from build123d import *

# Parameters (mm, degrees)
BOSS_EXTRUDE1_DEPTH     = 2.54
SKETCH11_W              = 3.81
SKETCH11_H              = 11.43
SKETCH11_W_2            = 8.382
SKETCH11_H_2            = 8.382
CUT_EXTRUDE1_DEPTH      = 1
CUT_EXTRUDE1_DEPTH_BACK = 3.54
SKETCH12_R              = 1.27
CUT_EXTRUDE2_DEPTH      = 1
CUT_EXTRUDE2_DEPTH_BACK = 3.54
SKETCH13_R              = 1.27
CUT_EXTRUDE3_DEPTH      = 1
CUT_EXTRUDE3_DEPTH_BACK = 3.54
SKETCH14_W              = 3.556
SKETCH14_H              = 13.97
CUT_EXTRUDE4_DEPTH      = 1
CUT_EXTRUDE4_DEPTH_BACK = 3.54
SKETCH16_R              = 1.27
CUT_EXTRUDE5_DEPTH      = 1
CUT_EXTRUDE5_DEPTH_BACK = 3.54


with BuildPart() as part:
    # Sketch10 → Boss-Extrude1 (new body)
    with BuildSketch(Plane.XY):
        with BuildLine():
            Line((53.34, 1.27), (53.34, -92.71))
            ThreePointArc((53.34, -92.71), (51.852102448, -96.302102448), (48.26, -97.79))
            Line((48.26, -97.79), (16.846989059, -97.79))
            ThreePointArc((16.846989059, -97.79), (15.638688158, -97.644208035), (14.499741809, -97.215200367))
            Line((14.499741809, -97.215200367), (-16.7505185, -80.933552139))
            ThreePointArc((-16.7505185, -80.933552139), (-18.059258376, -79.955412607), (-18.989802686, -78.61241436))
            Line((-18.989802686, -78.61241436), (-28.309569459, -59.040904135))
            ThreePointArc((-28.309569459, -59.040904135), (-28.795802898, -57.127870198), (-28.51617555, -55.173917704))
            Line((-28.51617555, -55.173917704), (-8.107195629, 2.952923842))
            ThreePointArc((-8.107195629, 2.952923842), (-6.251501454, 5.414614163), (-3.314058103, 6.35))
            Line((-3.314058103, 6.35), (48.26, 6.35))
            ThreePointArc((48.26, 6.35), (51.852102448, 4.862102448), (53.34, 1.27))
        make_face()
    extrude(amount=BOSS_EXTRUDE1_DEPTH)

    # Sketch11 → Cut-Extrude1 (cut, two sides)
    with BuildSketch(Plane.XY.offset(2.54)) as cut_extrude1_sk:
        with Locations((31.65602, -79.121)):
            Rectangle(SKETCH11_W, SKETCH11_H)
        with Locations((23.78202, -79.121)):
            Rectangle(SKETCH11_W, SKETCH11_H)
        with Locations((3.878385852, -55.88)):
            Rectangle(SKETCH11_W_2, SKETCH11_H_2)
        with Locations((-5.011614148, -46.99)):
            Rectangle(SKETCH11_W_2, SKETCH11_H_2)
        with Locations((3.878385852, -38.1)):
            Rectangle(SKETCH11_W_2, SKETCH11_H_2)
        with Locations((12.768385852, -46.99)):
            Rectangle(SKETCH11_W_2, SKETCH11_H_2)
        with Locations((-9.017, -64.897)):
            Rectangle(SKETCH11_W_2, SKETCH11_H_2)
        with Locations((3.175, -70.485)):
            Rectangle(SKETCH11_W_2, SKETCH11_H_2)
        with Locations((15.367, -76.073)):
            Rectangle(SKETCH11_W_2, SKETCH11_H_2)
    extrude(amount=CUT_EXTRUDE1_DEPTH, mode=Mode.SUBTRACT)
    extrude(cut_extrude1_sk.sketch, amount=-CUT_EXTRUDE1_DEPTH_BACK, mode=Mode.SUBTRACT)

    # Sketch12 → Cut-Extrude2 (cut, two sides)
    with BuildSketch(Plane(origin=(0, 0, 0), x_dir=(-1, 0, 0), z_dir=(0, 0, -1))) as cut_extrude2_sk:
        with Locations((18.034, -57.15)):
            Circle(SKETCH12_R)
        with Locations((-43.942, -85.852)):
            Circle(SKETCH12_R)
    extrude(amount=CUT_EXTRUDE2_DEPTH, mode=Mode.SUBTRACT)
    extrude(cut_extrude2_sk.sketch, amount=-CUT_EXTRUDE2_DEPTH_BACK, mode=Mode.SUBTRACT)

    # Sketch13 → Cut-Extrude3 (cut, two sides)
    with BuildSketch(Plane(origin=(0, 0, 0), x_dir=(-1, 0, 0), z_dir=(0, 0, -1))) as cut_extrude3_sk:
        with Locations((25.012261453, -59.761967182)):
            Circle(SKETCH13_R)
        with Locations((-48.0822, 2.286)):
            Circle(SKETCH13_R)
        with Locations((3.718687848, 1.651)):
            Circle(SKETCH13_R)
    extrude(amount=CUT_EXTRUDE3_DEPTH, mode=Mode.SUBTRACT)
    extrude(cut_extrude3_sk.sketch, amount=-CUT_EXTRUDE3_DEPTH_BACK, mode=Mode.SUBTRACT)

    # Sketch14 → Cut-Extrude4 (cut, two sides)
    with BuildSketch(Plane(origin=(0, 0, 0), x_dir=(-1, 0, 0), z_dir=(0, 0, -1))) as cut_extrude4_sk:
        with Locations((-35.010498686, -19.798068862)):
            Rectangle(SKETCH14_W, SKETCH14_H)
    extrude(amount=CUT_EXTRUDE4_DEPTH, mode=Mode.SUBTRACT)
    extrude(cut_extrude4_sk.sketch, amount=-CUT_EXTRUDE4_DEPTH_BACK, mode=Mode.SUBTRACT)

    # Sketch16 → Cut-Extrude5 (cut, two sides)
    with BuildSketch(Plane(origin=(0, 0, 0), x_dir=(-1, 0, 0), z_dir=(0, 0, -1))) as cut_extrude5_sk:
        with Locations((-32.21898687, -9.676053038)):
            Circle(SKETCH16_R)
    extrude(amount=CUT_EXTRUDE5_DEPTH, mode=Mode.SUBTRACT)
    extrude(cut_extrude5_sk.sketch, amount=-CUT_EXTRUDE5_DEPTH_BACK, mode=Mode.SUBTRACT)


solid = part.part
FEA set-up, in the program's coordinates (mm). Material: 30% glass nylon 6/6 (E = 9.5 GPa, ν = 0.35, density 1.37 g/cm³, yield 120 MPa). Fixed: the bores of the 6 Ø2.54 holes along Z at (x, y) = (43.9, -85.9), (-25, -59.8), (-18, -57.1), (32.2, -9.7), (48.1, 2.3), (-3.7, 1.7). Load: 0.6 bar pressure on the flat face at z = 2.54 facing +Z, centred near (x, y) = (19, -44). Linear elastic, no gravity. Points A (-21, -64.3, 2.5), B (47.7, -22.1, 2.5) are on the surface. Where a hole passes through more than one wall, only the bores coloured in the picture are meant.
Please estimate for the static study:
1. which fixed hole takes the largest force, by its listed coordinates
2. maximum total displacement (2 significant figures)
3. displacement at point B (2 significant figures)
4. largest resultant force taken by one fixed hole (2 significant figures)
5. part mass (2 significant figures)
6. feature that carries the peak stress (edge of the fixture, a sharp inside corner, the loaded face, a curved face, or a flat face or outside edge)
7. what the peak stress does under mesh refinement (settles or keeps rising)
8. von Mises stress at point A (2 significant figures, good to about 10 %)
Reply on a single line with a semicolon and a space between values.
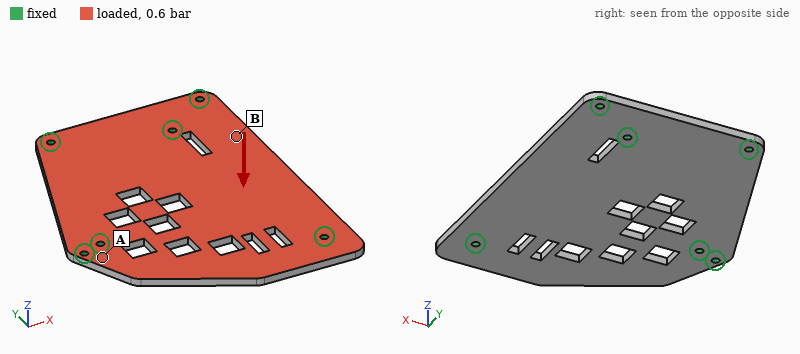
(-18, -57.1); 0.58 mm; 0.28 mm; 140 N; 23 g; edge of the fixture; keeps rising; 18 MPa
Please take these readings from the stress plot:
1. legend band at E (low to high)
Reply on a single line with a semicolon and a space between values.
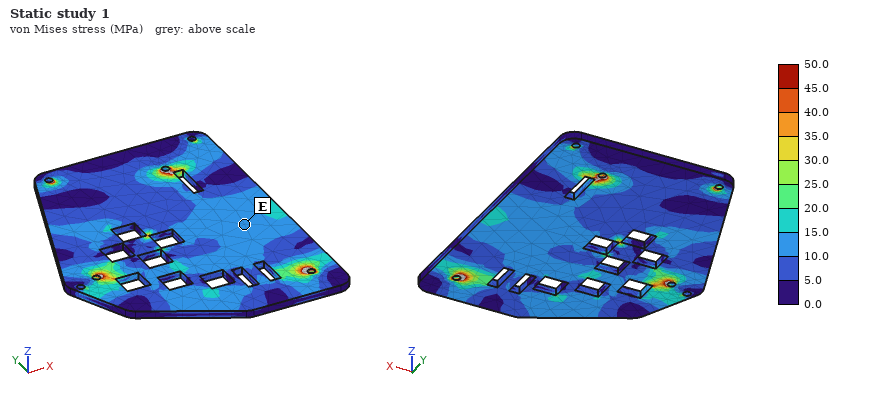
10.0 to 15.0 MPa
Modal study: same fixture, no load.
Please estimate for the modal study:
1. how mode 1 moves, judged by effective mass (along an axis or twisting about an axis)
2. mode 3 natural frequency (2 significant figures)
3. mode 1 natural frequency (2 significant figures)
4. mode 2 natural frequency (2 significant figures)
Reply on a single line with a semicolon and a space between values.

along Z; 1600 Hz; 1000 Hz; 1100 Hz
